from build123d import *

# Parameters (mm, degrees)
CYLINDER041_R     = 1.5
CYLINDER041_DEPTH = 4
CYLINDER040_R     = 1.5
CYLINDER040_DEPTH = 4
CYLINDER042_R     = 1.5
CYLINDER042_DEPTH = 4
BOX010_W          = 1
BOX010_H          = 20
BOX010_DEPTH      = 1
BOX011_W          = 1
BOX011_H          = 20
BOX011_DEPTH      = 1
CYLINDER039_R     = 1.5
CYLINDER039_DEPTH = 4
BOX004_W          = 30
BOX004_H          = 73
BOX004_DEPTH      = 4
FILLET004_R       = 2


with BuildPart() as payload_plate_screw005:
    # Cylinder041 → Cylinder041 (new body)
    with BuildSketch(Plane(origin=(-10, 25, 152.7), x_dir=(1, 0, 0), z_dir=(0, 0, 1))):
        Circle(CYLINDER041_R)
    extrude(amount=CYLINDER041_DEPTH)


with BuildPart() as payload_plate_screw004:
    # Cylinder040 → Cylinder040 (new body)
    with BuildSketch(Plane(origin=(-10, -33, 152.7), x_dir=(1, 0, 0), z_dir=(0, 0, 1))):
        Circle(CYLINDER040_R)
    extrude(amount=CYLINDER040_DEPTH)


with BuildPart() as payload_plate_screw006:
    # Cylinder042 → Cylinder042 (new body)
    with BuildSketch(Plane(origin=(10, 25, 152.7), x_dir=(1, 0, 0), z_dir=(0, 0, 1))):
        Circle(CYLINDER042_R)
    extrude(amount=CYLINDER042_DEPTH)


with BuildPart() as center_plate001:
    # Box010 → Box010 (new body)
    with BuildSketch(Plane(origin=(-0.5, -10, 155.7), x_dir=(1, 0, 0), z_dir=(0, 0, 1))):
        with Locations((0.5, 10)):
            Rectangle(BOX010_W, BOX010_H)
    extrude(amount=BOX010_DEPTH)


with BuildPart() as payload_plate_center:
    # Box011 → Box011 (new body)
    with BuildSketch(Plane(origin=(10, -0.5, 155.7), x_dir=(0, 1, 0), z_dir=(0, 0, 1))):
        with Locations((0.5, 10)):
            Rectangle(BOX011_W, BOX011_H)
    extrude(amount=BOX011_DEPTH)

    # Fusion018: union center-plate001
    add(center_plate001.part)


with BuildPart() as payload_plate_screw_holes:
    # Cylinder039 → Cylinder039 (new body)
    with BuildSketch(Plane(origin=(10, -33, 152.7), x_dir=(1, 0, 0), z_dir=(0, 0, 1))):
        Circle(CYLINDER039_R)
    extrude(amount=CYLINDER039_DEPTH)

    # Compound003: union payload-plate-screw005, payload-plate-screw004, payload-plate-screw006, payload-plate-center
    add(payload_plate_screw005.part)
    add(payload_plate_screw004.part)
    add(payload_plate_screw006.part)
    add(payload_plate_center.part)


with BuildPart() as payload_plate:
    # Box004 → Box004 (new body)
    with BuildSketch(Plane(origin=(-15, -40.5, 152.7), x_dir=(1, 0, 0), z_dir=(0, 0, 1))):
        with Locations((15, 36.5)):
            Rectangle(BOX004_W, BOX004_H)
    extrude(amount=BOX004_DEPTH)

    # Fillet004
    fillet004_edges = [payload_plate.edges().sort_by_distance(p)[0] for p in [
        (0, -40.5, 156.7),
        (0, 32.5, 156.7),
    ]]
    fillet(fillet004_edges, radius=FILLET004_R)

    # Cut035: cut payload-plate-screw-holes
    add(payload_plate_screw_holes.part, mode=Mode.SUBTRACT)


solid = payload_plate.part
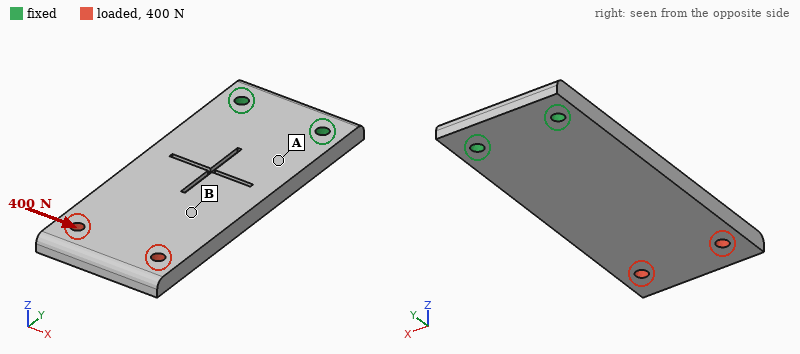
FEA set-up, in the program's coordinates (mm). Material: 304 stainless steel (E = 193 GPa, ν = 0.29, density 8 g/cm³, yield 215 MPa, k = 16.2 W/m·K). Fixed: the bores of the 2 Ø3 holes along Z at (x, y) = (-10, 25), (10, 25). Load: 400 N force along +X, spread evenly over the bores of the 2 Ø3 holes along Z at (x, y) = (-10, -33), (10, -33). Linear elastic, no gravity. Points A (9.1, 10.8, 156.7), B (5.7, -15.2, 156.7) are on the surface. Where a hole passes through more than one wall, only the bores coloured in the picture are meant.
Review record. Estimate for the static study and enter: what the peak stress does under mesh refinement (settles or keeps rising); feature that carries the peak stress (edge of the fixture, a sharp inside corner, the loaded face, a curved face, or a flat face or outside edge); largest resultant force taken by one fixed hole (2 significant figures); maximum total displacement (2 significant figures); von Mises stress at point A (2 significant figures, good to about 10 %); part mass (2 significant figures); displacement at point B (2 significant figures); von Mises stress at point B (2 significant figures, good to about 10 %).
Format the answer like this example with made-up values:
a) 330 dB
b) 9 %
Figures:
a) keeps rising
b) edge of the fixture
c) 1.1 kN
d) 23 µm
e) 18 MPa
f) 68 g
g) 11 µm
h) 8.8 MPa
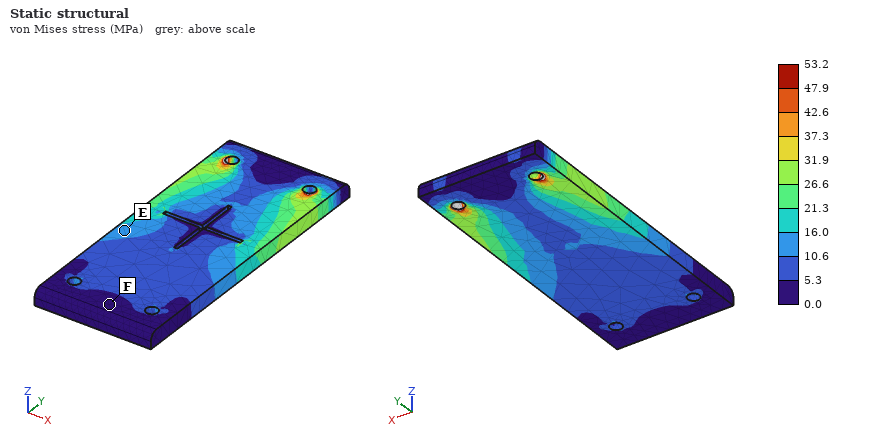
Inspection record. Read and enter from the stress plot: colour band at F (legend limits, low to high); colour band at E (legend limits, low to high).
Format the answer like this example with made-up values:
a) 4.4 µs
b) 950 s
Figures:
a) 0.0 to 5.3 MPa
b) 10.6 to 16.0 MPa
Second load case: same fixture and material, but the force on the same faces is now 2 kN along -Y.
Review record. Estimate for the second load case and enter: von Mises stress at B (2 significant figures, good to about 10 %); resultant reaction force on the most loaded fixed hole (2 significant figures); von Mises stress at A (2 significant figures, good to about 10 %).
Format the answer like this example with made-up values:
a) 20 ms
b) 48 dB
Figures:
a) 16 MPa
b) 1.0 kN
c) 17 MPa
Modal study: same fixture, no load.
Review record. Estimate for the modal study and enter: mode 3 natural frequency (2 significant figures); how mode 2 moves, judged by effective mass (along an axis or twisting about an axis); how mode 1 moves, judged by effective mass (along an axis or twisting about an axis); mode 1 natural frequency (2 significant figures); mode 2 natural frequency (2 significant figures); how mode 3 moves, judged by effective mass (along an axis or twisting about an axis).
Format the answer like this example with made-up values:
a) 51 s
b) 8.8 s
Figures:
a) 4500 Hz
b) twisting about Y
c) along Z
d) 730 Hz
e) 3300 Hz
f) along Z
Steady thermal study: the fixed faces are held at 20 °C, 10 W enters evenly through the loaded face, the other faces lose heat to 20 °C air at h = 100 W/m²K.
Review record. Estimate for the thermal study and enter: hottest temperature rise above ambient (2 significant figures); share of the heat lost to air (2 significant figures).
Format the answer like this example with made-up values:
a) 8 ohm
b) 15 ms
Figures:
a) 71 K
b) 96 %
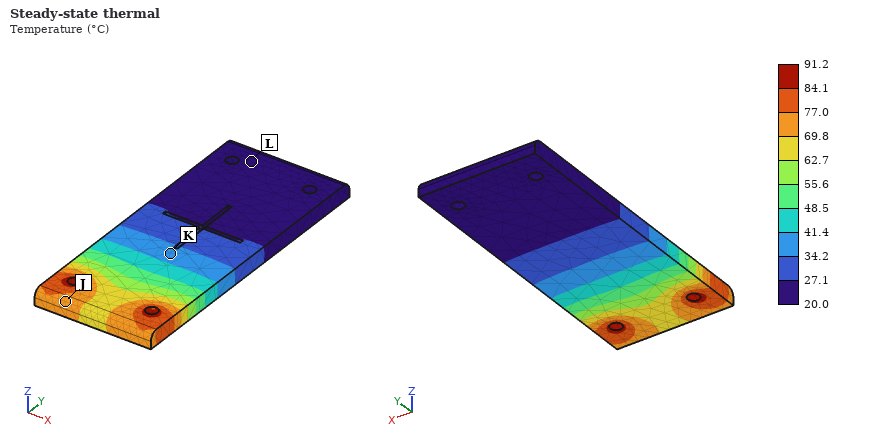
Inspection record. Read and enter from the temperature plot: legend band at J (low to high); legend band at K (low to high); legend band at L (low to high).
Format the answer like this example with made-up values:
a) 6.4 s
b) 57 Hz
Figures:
a) 69.8 to 77.0 °C
b) 34.2 to 41.4 °C
c) 20.0 to 27.1 °C
